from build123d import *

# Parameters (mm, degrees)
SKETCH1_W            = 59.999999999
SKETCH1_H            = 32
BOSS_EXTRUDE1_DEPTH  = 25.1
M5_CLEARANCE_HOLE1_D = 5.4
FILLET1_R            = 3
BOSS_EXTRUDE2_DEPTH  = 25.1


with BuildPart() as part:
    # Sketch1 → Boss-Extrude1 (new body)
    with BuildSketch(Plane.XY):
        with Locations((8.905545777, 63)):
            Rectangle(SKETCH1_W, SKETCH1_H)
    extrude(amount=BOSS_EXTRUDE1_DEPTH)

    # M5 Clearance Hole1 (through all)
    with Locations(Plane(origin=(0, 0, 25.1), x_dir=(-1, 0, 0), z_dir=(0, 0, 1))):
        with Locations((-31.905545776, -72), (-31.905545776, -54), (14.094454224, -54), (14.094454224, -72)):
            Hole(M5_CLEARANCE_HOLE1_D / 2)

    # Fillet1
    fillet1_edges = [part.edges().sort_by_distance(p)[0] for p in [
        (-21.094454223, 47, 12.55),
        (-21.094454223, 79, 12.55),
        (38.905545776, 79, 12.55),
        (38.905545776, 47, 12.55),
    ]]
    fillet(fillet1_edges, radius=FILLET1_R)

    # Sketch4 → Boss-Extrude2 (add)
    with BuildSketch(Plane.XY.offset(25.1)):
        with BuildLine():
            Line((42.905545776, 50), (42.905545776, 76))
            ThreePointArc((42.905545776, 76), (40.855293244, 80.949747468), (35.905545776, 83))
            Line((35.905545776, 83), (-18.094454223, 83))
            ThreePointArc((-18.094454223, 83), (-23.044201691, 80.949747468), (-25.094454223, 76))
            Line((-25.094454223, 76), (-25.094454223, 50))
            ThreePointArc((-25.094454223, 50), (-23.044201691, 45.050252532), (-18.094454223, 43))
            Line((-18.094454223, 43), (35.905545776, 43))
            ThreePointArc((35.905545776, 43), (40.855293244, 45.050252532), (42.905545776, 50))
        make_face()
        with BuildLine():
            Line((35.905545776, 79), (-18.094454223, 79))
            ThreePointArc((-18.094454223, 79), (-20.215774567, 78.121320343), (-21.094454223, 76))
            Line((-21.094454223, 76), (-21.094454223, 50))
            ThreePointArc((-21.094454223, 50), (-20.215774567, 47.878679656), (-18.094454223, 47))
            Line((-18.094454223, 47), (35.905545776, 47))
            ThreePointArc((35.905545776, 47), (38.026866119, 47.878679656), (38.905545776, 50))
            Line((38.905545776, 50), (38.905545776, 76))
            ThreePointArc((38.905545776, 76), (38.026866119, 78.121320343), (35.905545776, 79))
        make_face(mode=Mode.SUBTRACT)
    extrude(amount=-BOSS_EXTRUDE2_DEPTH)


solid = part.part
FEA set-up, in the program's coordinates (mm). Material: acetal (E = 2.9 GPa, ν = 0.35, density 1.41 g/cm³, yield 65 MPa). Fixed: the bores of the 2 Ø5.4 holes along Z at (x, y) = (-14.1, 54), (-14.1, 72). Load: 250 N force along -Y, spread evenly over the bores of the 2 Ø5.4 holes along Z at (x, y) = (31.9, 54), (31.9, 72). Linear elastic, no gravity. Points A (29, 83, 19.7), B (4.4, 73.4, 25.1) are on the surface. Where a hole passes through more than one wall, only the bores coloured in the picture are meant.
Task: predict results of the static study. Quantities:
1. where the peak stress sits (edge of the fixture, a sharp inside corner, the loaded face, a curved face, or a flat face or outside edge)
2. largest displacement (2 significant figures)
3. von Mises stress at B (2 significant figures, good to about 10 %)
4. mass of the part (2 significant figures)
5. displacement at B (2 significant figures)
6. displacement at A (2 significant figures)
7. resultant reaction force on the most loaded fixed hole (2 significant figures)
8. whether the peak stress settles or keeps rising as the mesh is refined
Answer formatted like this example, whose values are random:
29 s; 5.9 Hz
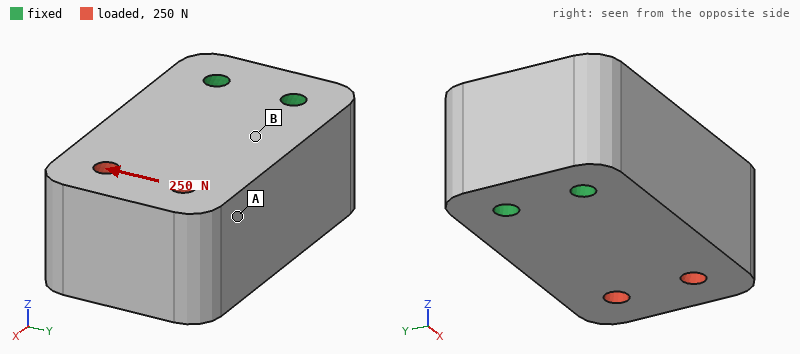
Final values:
edge of the fixture; 55 µm; 0.74 MPa; 92 g; 15 µm; 44 µm; 530 N; keeps rising
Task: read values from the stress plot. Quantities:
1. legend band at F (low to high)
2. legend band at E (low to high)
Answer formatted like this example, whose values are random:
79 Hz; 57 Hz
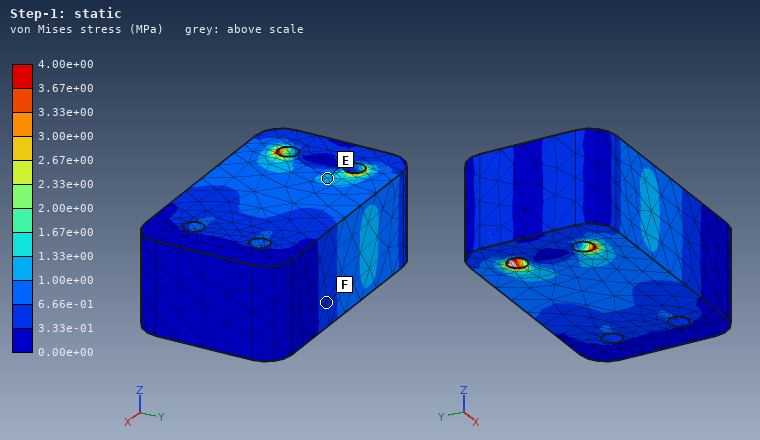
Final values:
3.33e-01 to 6.66e-01 MPa; 1.00e+00 to 1.33e+00 MPa
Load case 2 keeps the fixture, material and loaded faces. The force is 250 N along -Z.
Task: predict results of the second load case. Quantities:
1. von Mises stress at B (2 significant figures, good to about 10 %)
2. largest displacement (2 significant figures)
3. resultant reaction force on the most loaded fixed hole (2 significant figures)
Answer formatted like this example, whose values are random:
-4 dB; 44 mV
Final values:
1.7 MPa; 93 µm; 130 N
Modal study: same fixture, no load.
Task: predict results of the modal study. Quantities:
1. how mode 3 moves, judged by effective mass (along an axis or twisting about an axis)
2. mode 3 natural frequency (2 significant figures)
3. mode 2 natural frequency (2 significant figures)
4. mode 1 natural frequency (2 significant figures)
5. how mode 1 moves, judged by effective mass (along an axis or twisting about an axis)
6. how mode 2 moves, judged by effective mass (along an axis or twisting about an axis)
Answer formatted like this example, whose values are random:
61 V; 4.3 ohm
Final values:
twisting about X; 3400 Hz; 1900 Hz; 1600 Hz; along Z; along Y
